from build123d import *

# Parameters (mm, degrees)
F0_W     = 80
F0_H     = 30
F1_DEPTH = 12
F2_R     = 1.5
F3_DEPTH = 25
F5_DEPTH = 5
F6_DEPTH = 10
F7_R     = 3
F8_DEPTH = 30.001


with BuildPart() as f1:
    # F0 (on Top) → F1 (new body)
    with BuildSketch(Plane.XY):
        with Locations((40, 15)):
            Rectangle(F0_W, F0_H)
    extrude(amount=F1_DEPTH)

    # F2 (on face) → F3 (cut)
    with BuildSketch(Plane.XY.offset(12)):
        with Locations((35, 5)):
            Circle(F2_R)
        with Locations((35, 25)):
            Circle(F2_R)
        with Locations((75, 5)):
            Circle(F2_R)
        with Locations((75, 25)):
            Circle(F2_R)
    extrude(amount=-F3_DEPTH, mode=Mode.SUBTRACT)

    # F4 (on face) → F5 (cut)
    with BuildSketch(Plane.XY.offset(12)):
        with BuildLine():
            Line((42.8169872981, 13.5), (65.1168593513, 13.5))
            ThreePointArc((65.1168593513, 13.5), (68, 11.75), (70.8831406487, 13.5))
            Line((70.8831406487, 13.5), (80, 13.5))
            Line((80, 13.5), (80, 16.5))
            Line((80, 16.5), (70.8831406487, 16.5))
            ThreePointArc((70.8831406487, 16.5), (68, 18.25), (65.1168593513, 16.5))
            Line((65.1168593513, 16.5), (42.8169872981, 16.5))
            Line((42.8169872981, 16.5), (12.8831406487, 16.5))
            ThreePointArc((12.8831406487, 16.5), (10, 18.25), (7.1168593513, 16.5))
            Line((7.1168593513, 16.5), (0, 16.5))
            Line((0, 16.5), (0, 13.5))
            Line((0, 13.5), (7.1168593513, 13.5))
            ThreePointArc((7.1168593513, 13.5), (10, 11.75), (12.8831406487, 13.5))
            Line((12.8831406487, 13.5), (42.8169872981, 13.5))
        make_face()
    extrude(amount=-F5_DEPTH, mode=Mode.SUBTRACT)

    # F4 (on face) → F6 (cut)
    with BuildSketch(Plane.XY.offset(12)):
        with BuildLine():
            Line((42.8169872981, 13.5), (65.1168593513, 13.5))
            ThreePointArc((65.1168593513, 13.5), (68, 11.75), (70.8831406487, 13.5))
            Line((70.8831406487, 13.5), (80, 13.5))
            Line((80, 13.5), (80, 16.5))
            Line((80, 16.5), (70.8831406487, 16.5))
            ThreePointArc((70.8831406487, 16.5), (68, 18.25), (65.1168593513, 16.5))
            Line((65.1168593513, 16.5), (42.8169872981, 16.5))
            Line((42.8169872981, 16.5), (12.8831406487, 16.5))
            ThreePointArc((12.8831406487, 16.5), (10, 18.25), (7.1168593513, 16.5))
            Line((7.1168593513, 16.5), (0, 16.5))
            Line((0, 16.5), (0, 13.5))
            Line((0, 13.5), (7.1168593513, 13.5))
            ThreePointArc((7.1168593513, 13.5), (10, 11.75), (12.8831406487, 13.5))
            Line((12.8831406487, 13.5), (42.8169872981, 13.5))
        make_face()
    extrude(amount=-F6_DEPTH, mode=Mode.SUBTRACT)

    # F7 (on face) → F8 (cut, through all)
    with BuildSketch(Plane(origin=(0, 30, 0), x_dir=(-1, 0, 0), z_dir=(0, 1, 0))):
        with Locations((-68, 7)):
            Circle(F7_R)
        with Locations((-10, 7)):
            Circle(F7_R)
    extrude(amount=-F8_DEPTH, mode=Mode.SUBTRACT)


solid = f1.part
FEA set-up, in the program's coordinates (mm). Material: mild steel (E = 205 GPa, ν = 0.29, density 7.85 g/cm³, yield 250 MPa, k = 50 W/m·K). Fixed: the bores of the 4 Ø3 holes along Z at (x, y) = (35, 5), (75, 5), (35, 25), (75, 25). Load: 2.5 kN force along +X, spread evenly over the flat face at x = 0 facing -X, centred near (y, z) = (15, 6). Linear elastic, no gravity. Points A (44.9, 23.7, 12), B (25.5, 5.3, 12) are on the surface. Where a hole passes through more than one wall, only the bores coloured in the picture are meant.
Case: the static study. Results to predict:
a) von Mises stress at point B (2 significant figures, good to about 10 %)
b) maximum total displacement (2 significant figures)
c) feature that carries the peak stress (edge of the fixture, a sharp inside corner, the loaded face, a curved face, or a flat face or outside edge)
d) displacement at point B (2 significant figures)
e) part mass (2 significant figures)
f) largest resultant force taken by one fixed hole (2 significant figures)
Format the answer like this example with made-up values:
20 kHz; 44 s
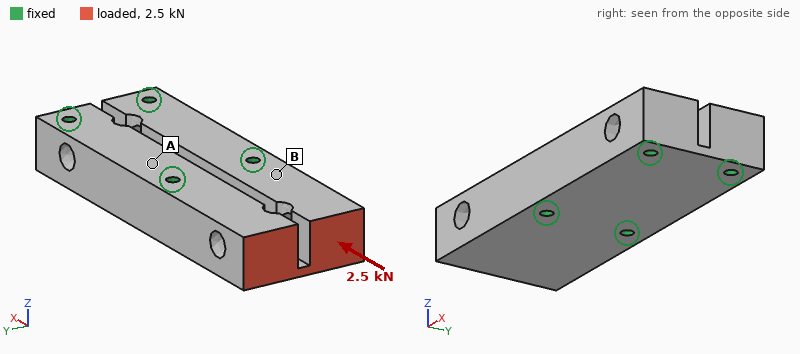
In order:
8.6 MPa; 2.2 µm; a curved face; 0.44 µm; 190 g; 1.2 kN
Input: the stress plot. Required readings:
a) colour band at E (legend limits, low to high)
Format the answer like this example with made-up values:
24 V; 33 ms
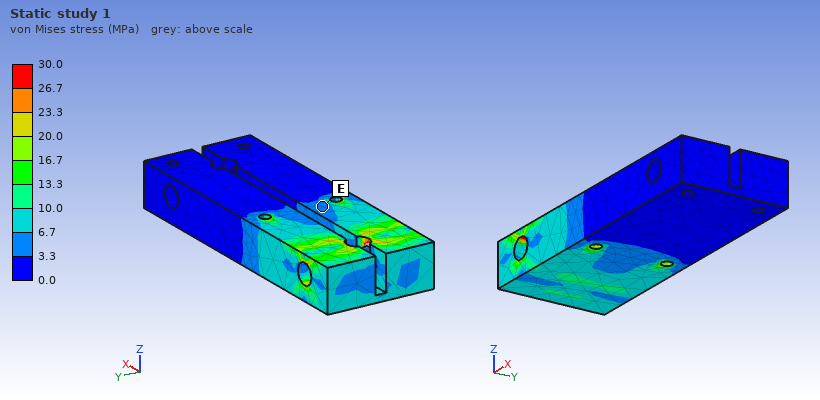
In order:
3.3 to 6.7 MPa
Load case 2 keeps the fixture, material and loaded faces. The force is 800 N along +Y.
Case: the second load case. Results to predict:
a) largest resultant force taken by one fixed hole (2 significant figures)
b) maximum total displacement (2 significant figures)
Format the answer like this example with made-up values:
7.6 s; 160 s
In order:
1.2 kN; 9.1 µm
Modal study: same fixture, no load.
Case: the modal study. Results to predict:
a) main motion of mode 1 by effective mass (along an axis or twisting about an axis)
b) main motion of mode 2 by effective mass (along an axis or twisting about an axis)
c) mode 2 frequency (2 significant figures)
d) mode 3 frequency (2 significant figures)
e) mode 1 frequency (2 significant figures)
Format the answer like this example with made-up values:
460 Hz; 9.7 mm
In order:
along Z; along Y; 10 kHz; 15 kHz; 7300 Hz
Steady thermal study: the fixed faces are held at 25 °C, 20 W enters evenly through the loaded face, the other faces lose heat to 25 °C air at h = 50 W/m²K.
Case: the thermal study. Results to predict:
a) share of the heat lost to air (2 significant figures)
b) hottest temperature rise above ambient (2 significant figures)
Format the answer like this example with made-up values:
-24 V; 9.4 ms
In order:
22 %; 45 K
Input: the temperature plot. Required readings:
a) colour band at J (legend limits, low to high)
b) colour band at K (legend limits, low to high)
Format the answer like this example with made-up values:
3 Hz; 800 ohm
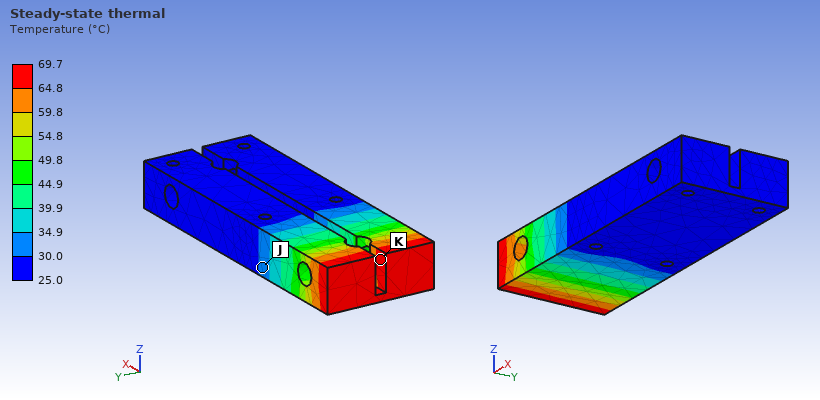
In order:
30.0 to 34.9 °C; 64.8 to 69.7 °C
